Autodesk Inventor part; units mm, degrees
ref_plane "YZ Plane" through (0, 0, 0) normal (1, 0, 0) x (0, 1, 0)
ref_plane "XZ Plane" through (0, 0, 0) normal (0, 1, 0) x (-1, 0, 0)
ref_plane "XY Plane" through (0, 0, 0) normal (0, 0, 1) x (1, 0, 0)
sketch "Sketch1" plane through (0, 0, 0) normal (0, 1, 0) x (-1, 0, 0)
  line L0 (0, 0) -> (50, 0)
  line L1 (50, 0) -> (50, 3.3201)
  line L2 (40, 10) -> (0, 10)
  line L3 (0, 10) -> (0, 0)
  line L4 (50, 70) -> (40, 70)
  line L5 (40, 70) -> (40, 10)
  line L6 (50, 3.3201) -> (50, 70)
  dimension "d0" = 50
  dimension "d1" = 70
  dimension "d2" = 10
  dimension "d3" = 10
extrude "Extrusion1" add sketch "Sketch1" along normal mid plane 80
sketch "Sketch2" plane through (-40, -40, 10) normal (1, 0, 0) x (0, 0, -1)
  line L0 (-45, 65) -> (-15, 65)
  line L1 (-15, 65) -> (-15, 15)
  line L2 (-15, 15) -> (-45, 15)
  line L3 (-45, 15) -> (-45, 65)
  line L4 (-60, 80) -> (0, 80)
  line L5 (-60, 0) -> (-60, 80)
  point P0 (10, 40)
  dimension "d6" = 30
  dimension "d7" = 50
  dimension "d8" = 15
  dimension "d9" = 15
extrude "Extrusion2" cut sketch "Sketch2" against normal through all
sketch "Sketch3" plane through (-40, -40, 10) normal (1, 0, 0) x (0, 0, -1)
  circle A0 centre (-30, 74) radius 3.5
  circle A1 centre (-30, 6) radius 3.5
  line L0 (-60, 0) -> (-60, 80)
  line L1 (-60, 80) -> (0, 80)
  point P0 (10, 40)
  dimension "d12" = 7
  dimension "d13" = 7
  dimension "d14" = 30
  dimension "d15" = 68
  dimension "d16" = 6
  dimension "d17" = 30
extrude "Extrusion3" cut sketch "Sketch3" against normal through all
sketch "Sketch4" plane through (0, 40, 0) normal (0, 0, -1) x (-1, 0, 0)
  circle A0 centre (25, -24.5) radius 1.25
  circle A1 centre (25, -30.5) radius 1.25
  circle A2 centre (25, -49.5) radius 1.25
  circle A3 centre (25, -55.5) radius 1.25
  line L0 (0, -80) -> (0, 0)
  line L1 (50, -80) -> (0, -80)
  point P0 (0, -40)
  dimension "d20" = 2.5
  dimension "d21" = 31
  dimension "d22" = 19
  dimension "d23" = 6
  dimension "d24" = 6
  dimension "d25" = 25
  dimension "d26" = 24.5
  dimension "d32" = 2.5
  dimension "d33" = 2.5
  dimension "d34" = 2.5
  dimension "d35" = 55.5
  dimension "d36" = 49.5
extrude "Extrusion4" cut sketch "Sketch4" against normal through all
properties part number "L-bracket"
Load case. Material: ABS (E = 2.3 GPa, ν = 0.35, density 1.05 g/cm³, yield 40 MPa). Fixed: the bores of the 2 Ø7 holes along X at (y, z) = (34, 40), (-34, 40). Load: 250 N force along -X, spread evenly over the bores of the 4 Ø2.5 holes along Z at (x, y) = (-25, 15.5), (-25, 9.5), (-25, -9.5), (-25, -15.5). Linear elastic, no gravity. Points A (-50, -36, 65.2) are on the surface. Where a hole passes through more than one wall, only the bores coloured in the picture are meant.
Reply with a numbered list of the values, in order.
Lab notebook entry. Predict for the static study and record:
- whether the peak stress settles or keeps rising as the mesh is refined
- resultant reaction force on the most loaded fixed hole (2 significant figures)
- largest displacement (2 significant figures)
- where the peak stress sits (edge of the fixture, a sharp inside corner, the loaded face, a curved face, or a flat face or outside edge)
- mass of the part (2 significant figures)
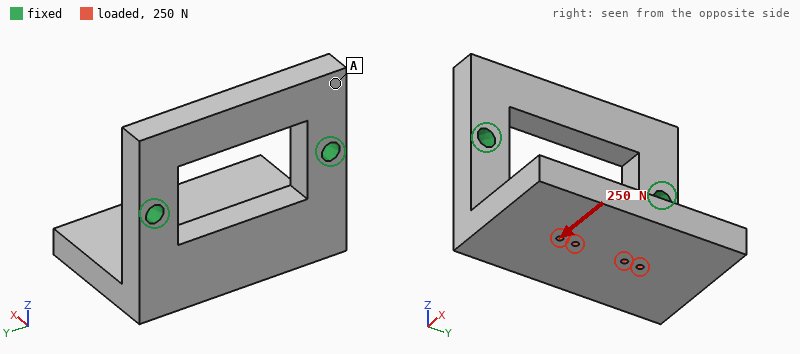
1. keeps rising
2. 130 N
3. 1.2 mm
4. edge of the fixture
5. 76 g
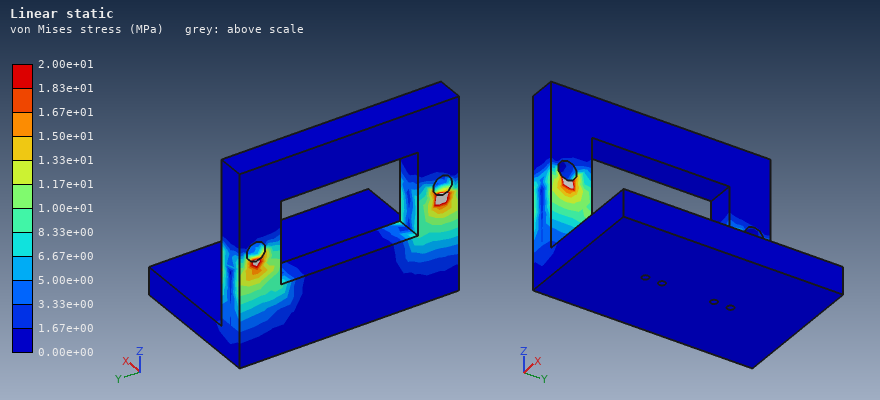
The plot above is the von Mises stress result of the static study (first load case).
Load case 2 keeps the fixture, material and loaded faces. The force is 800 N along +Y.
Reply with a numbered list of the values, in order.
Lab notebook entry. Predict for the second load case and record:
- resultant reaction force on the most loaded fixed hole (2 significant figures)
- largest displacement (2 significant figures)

1. 550 N
2. 0.78 mm
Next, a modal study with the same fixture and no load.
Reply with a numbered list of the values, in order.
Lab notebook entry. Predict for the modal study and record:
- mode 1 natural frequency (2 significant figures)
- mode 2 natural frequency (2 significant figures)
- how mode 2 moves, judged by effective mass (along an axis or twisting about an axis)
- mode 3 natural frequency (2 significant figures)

1. 350 Hz
2. 810 Hz
3. along Y
4. 1100 Hz
